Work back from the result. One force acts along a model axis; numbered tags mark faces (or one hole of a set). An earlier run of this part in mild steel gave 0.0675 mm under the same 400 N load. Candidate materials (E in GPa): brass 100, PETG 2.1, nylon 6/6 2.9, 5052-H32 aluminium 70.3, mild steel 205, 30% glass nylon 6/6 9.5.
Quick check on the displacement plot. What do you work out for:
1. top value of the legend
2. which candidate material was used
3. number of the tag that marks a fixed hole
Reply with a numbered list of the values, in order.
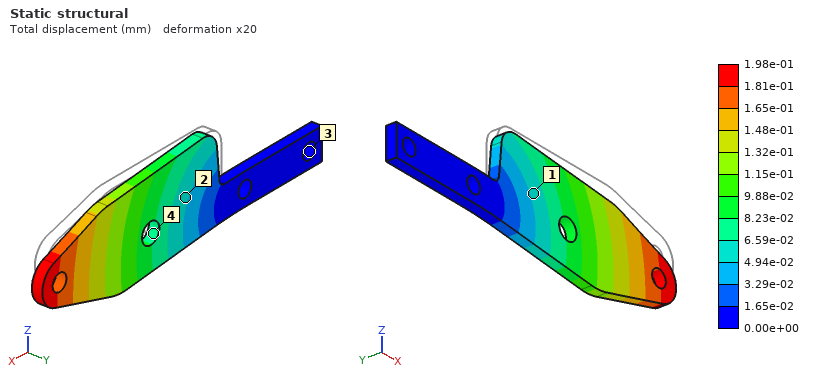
1. 1.98e-01 mm
2. 5052-H32 aluminium
3. 3
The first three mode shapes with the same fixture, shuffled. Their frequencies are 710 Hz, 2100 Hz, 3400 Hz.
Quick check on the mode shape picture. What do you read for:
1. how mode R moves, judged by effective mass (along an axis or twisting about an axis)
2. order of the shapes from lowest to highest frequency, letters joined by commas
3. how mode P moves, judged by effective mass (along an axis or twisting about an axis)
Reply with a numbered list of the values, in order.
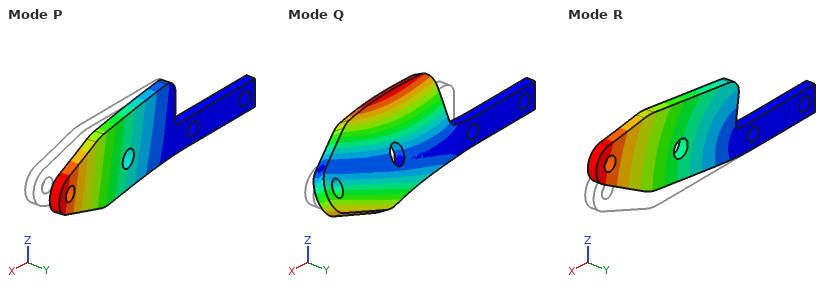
1. along Z
2. P, R, Q
3. along Y
